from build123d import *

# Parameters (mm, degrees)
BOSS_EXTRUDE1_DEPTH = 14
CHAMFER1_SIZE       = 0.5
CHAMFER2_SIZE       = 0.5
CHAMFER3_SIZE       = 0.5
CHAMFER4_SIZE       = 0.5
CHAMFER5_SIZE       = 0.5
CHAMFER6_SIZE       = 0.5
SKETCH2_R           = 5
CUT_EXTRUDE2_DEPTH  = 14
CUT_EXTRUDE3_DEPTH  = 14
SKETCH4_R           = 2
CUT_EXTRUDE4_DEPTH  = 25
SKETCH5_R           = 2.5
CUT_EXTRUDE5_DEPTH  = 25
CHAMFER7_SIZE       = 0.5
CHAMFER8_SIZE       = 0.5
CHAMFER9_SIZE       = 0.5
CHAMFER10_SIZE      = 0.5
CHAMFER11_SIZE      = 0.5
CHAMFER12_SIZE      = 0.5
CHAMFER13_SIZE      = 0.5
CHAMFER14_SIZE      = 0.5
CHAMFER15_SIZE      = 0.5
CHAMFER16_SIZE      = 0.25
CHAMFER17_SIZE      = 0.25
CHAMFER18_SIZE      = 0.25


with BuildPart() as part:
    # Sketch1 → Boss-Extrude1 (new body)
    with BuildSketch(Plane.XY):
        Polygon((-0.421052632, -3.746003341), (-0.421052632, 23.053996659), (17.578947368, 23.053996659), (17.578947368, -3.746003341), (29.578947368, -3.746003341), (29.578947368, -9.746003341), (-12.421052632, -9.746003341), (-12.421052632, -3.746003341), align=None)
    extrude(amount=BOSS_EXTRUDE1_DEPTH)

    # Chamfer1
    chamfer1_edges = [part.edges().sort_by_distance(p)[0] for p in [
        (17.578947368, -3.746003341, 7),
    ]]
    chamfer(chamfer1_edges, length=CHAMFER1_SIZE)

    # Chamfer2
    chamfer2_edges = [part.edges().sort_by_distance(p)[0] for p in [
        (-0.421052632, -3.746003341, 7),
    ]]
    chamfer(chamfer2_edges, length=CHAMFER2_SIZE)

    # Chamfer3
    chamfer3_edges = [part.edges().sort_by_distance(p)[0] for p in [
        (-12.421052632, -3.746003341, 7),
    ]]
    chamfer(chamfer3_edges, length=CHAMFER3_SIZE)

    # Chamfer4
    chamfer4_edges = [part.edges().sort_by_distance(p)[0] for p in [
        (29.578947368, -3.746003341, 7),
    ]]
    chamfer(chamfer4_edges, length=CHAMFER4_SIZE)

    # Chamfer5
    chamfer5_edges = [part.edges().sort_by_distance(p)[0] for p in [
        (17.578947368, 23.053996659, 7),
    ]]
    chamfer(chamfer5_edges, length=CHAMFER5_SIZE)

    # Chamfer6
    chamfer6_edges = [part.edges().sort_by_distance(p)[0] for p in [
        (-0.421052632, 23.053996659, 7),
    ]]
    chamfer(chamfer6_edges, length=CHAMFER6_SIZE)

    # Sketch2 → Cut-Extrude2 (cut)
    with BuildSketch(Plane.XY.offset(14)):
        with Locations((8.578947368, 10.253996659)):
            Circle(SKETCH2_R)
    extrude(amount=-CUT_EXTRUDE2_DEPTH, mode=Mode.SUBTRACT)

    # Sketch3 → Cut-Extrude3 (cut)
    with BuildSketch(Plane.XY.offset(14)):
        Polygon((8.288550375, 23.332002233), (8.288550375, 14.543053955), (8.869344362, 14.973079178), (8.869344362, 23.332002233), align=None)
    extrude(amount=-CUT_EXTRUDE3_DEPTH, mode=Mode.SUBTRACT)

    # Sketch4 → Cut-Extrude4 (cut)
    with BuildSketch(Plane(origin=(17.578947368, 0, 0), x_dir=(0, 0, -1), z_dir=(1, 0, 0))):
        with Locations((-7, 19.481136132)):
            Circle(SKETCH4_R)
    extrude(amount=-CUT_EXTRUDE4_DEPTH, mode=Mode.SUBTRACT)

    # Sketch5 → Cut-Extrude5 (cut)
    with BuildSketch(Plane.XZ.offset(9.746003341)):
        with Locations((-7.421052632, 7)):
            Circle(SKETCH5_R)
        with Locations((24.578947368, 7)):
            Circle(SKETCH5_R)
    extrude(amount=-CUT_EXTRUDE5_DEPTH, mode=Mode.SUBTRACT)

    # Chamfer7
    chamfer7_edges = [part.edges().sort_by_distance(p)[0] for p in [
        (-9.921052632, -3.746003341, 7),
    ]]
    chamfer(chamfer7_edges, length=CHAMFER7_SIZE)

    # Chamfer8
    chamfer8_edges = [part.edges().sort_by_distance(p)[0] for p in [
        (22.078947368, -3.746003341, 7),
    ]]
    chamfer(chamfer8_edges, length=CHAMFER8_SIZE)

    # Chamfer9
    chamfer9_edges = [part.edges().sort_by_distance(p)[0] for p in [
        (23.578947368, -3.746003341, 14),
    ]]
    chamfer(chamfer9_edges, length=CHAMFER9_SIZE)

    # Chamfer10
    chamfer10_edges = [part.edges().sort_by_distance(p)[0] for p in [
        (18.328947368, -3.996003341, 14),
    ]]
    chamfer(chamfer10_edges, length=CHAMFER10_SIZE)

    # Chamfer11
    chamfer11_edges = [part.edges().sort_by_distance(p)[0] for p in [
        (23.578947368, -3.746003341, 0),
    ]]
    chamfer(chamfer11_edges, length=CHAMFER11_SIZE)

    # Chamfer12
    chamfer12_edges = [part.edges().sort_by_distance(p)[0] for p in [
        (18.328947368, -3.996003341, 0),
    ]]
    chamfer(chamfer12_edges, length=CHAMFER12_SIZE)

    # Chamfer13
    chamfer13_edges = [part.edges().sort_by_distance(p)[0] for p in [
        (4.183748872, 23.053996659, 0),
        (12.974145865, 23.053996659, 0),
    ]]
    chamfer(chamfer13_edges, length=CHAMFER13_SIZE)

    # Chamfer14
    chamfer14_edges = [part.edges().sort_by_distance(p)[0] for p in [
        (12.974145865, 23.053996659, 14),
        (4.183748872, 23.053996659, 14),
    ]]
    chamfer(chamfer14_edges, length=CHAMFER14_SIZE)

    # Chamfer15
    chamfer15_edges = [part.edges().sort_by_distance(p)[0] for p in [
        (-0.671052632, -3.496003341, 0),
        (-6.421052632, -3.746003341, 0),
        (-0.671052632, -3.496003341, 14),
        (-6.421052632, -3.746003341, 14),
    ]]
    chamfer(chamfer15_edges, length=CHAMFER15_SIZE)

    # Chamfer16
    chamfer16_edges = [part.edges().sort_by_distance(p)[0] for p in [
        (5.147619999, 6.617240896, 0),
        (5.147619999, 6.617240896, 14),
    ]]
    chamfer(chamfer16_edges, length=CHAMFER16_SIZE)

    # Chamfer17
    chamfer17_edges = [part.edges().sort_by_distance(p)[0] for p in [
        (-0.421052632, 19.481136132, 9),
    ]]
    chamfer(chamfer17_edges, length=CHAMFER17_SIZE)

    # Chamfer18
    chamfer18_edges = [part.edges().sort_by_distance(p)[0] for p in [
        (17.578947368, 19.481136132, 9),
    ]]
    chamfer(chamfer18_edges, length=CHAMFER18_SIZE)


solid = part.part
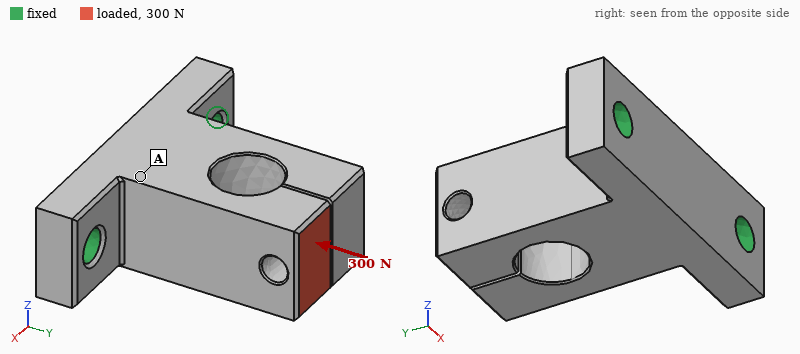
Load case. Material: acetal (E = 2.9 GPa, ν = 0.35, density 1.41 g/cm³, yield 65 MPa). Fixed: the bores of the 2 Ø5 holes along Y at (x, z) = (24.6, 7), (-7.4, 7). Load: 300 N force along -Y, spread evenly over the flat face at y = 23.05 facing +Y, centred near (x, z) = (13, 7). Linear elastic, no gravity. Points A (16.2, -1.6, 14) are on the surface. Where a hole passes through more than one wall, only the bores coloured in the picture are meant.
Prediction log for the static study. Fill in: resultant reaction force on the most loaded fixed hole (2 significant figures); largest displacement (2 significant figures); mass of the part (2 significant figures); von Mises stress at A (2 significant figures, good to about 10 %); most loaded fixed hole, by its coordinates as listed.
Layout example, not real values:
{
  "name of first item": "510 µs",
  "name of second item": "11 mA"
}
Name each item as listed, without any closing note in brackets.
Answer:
{
  "resultant reaction force on the most loaded fixed hole": "210 N",
  "largest displacement": "0.36 mm",
  "mass of the part": "12 g",
  "von Mises stress at A": "4.1 MPa",
  "most loaded fixed hole, by its coordinates as listed": "(24.6, 7)"
}
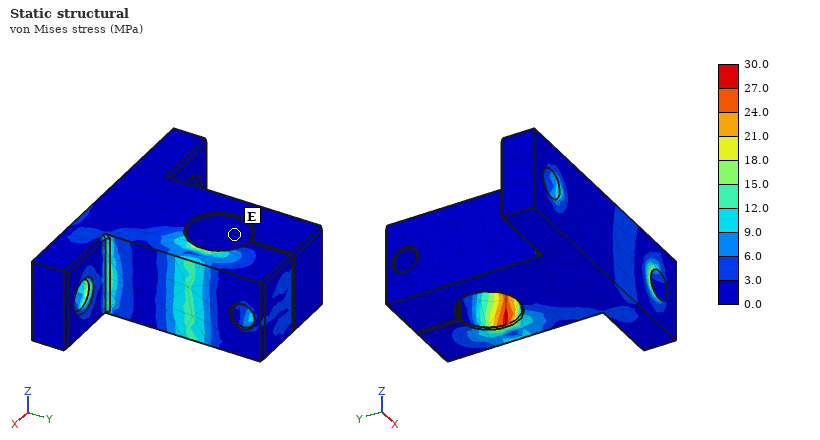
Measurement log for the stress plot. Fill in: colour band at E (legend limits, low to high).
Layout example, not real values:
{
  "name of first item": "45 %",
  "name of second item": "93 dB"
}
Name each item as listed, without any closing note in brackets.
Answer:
{
  "colour band at E": "0.0 to 3.0 MPa"
}
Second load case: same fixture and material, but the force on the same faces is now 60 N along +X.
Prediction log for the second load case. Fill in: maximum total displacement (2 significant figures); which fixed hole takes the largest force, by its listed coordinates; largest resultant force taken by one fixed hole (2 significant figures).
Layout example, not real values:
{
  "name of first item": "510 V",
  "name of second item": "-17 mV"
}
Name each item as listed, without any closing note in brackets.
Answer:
{
  "maximum total displacement": "0.50 mm",
  "which fixed hole takes the largest force, by its listed coordinates": "(-7.4, 7)",
  "largest resultant force taken by one fixed hole": "85 N"
}
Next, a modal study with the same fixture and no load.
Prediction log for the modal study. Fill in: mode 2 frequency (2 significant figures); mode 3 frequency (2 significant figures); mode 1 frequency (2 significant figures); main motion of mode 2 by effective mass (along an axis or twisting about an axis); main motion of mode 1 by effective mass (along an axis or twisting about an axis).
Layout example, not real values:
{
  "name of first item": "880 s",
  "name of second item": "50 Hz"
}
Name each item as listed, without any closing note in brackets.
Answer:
{
  "mode 2 frequency": "1900 Hz",
  "mode 3 frequency": "2200 Hz",
  "mode 1 frequency": "1400 Hz",
  "main motion of mode 2 by effective mass": "along X",
  "main motion of mode 1 by effective mass": "along Z"
}
